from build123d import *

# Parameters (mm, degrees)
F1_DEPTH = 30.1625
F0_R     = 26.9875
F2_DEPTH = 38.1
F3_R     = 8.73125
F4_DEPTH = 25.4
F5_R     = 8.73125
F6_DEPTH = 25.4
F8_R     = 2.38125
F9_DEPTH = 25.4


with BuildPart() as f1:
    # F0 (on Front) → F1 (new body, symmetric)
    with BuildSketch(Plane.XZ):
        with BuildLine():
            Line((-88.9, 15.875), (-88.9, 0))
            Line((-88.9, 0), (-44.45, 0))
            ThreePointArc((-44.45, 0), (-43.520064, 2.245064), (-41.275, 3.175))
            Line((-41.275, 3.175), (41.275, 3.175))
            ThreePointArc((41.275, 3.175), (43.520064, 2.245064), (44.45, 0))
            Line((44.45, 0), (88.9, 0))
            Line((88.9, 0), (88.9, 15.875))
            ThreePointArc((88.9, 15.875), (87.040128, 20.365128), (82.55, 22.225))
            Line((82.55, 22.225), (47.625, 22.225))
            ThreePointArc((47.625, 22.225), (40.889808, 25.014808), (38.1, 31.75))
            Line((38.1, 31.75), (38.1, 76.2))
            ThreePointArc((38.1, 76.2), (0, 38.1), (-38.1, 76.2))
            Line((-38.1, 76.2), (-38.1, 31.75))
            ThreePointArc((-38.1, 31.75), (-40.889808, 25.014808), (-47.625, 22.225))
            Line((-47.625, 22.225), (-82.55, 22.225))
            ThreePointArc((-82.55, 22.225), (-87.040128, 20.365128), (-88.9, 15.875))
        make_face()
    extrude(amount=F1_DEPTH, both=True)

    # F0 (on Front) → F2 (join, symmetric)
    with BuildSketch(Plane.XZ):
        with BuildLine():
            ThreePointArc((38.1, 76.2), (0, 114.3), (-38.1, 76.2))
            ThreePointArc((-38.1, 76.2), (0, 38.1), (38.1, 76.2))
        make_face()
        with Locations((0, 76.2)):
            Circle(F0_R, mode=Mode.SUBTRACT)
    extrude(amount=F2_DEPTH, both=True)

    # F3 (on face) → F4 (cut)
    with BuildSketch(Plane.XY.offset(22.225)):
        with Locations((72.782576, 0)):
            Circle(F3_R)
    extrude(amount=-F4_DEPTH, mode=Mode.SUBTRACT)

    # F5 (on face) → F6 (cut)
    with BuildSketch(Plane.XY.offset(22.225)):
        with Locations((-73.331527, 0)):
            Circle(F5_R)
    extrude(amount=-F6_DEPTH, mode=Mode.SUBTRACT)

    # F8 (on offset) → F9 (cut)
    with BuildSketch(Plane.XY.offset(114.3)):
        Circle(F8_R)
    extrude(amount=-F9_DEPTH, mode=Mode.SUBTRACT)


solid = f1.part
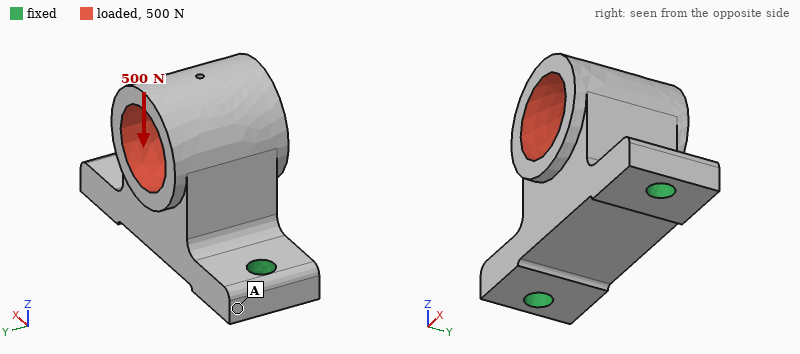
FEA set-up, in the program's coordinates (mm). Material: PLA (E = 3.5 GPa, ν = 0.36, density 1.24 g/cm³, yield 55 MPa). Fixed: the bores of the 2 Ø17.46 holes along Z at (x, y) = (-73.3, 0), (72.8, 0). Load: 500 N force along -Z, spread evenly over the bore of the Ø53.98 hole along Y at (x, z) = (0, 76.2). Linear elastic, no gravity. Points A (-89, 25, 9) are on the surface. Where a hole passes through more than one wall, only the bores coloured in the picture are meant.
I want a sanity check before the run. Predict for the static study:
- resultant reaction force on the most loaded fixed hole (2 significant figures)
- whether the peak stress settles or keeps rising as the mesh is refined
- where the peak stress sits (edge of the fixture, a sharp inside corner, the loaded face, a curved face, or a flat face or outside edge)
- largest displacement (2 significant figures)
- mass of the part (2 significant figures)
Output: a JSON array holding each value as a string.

["290 N", "keeps rising", "edge of the fixture", "23 µm", "610 g"]
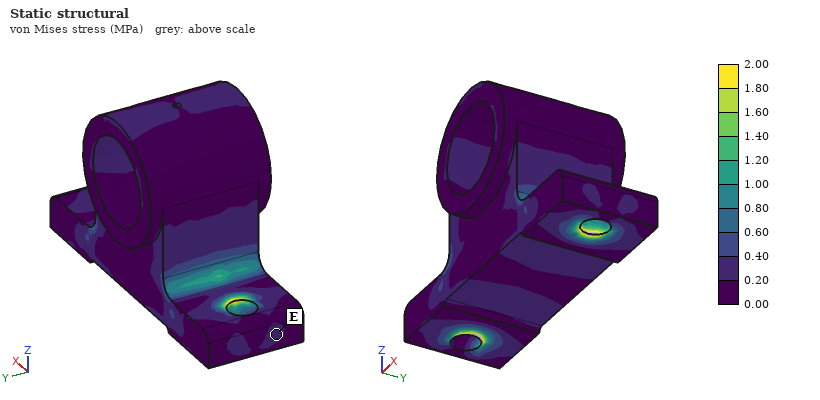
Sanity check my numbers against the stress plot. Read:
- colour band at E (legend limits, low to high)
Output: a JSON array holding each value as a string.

["0.20 to 0.40 MPa"]
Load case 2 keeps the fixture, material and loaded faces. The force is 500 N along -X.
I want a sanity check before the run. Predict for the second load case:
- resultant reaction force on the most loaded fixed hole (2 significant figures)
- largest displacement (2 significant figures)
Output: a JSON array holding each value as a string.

["380 N", "75 µm"]
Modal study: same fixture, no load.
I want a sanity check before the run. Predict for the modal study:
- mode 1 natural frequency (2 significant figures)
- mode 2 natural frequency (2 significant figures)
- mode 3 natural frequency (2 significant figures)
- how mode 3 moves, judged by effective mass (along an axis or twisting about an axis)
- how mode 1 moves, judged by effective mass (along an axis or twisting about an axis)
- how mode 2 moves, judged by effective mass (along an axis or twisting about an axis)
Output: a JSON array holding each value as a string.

["480 Hz", "970 Hz", "1300 Hz", "along Z", "along Y", "along X"]
